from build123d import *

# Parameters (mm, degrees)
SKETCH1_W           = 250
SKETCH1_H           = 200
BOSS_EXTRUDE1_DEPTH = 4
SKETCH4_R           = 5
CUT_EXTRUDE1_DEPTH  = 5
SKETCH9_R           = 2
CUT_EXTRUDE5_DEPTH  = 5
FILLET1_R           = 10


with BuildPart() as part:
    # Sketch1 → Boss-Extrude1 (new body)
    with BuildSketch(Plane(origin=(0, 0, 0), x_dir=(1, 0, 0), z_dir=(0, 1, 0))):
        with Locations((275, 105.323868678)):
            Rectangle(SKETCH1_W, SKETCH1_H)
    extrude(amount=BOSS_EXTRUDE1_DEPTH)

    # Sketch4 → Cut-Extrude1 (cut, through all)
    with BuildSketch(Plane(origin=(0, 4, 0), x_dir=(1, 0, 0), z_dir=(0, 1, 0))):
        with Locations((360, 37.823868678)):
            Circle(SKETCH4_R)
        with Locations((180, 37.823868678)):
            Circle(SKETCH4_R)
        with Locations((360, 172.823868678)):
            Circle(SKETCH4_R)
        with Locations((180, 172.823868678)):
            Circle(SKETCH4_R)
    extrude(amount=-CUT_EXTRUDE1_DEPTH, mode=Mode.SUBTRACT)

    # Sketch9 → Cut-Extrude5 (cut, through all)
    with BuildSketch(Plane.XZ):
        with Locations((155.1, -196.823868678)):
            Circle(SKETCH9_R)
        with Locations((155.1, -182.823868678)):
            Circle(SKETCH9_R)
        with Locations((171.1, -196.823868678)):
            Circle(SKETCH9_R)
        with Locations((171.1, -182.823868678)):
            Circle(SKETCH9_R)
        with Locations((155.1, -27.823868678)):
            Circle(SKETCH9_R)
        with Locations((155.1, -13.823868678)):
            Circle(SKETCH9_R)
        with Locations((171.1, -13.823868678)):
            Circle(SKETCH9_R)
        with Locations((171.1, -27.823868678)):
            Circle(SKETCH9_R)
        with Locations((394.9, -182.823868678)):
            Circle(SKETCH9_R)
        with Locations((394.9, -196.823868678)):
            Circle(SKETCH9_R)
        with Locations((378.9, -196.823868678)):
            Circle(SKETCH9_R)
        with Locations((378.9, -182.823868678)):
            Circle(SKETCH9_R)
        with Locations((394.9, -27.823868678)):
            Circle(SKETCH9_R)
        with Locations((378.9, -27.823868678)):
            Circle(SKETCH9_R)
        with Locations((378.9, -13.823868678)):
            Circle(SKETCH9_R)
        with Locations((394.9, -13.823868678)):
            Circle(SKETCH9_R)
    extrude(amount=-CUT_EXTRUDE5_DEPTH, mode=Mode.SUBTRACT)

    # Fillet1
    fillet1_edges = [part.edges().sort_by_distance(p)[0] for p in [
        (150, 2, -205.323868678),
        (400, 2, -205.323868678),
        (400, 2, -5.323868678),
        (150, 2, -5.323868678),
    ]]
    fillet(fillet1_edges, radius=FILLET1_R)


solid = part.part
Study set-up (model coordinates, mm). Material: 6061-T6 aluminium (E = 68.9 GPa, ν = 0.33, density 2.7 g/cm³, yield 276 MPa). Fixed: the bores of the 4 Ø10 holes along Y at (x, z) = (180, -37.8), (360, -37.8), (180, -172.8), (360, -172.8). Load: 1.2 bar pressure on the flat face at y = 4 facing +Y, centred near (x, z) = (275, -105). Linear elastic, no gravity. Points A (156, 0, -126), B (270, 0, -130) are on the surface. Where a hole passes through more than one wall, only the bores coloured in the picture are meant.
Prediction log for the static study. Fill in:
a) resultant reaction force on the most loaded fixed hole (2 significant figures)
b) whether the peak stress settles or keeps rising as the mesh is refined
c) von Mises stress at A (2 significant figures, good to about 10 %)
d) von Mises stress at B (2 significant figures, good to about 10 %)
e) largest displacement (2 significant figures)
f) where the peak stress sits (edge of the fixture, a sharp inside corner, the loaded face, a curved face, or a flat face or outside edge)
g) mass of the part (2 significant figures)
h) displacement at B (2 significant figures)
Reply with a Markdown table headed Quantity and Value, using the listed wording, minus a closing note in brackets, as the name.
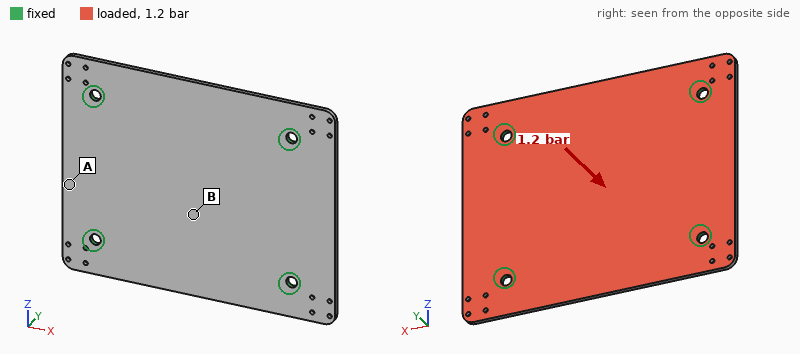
| Quantity | Value |
|---|---|
| resultant reaction force on the most loaded fixed hole | 1.5 kN |
| whether the peak stress settles or keeps rising as the mesh is refined | keeps rising |
| von Mises stress at A | 22 MPa |
| von Mises stress at B | 57 MPa |
| largest displacement | 1.2 mm |
| where the peak stress sits | edge of the fixture |
| mass of the part | 530 g |
| displacement at B | 1.2 mm |
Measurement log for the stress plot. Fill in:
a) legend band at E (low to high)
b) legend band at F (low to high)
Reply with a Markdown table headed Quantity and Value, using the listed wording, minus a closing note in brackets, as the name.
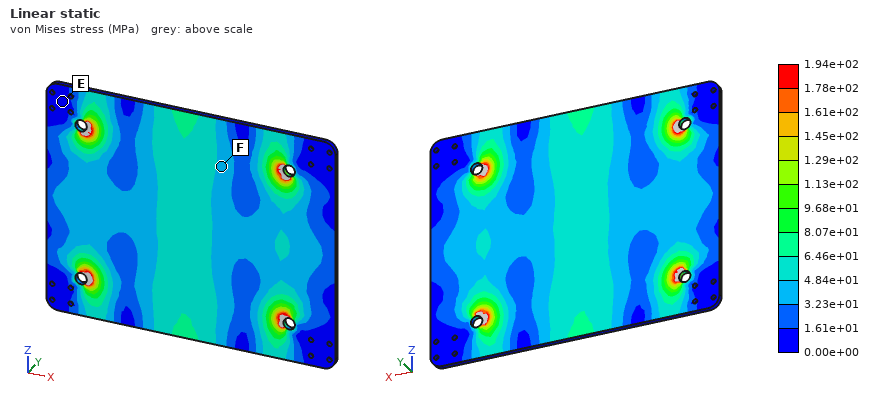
| Quantity | Value |
|---|---|
| legend band at E | 0.00e+00 to 1.61e+01 MPa |
| legend band at F | 3.23e+01 to 4.84e+01 MPa |
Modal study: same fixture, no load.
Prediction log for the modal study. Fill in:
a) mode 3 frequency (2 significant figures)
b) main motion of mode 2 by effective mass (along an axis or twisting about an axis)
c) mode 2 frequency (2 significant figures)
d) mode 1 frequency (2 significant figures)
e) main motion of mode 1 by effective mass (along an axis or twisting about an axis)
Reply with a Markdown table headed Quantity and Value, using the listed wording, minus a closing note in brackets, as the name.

| Quantity | Value |
|---|---|
| mode 3 frequency | 930 Hz |
| main motion of mode 2 by effective mass | twisting about X |
| mode 2 frequency | 730 Hz |
| mode 1 frequency | 560 Hz |
| main motion of mode 1 by effective mass | along Y |
